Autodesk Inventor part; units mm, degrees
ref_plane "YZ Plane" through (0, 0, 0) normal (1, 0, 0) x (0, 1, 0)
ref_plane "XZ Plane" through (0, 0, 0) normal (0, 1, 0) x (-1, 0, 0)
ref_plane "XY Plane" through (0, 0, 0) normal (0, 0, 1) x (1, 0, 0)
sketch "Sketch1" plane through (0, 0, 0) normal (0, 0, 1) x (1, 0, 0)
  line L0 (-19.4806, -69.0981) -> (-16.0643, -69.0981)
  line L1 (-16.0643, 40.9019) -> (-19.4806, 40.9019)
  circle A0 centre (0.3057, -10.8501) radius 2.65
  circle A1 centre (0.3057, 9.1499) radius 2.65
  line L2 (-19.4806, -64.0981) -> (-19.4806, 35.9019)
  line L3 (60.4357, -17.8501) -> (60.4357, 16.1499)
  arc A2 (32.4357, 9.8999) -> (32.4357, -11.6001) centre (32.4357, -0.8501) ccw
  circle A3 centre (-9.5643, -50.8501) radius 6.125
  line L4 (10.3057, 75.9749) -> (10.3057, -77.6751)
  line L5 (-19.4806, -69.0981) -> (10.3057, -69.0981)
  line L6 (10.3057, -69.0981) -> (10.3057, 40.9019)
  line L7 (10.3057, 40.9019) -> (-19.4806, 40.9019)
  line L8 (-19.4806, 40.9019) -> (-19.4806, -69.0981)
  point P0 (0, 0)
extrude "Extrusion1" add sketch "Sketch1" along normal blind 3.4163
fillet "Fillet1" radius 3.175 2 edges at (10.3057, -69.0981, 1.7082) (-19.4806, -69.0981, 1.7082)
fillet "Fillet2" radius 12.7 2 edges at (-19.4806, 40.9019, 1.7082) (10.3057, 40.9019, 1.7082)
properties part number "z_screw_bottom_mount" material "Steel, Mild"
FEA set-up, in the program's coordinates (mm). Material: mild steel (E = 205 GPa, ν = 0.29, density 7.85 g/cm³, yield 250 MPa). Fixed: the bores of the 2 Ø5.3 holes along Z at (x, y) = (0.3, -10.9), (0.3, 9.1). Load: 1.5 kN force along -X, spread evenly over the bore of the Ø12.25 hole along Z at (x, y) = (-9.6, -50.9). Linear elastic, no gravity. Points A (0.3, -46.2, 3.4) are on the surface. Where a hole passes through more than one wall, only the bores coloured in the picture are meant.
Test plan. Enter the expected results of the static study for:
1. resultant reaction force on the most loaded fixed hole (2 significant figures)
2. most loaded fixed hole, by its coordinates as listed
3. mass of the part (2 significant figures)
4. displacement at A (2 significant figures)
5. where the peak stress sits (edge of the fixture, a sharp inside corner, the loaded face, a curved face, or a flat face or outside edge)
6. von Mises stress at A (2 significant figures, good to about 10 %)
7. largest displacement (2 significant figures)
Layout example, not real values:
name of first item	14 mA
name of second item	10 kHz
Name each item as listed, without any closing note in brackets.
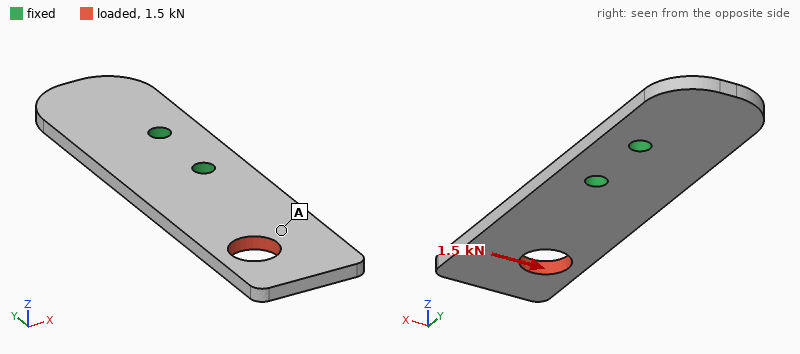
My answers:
resultant reaction force on the most loaded fixed hole	3.7 kN
most loaded fixed hole, by its coordinates as listed	(0.3, -10.9)
mass of the part	82 g
displacement at A	45 µm
where the peak stress sits	edge of the fixture
von Mises stress at A	30 MPa
largest displacement	82 µm
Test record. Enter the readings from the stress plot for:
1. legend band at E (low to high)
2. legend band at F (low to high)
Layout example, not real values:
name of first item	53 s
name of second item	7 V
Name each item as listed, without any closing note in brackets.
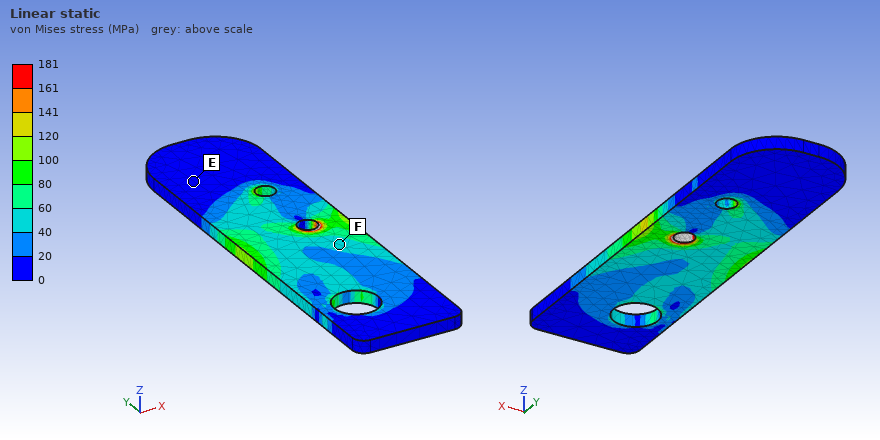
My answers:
legend band at E	0 to 20 MPa
legend band at F	40 to 60 MPa
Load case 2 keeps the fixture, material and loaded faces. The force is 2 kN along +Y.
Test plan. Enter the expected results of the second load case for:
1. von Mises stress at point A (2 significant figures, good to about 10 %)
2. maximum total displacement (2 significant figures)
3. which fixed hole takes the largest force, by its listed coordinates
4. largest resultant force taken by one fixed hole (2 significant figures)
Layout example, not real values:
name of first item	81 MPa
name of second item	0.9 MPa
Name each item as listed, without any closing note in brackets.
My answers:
von Mises stress at point A	19 MPa
maximum total displacement	25 µm
which fixed hole takes the largest force, by its listed coordinates	(0.3, -10.9)
largest resultant force taken by one fixed hole	1.5 kN
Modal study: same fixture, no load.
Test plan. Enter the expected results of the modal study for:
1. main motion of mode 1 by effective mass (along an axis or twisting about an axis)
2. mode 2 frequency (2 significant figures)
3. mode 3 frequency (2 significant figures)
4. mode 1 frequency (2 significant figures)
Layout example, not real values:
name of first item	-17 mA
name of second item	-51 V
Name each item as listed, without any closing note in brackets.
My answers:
main motion of mode 1 by effective mass	along Z
mode 2 frequency	3000 Hz
mode 3 frequency	3100 Hz
mode 1 frequency	870 Hz
